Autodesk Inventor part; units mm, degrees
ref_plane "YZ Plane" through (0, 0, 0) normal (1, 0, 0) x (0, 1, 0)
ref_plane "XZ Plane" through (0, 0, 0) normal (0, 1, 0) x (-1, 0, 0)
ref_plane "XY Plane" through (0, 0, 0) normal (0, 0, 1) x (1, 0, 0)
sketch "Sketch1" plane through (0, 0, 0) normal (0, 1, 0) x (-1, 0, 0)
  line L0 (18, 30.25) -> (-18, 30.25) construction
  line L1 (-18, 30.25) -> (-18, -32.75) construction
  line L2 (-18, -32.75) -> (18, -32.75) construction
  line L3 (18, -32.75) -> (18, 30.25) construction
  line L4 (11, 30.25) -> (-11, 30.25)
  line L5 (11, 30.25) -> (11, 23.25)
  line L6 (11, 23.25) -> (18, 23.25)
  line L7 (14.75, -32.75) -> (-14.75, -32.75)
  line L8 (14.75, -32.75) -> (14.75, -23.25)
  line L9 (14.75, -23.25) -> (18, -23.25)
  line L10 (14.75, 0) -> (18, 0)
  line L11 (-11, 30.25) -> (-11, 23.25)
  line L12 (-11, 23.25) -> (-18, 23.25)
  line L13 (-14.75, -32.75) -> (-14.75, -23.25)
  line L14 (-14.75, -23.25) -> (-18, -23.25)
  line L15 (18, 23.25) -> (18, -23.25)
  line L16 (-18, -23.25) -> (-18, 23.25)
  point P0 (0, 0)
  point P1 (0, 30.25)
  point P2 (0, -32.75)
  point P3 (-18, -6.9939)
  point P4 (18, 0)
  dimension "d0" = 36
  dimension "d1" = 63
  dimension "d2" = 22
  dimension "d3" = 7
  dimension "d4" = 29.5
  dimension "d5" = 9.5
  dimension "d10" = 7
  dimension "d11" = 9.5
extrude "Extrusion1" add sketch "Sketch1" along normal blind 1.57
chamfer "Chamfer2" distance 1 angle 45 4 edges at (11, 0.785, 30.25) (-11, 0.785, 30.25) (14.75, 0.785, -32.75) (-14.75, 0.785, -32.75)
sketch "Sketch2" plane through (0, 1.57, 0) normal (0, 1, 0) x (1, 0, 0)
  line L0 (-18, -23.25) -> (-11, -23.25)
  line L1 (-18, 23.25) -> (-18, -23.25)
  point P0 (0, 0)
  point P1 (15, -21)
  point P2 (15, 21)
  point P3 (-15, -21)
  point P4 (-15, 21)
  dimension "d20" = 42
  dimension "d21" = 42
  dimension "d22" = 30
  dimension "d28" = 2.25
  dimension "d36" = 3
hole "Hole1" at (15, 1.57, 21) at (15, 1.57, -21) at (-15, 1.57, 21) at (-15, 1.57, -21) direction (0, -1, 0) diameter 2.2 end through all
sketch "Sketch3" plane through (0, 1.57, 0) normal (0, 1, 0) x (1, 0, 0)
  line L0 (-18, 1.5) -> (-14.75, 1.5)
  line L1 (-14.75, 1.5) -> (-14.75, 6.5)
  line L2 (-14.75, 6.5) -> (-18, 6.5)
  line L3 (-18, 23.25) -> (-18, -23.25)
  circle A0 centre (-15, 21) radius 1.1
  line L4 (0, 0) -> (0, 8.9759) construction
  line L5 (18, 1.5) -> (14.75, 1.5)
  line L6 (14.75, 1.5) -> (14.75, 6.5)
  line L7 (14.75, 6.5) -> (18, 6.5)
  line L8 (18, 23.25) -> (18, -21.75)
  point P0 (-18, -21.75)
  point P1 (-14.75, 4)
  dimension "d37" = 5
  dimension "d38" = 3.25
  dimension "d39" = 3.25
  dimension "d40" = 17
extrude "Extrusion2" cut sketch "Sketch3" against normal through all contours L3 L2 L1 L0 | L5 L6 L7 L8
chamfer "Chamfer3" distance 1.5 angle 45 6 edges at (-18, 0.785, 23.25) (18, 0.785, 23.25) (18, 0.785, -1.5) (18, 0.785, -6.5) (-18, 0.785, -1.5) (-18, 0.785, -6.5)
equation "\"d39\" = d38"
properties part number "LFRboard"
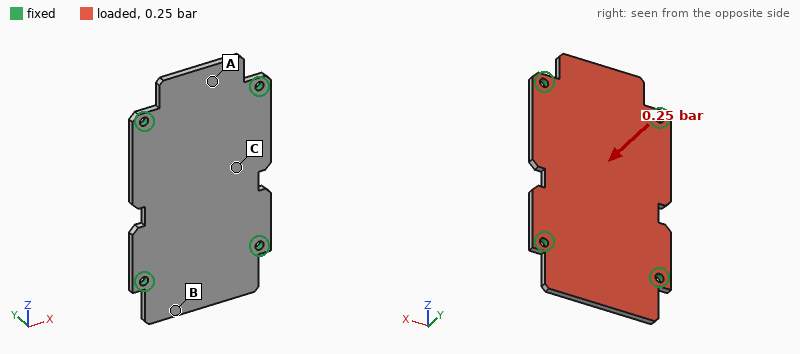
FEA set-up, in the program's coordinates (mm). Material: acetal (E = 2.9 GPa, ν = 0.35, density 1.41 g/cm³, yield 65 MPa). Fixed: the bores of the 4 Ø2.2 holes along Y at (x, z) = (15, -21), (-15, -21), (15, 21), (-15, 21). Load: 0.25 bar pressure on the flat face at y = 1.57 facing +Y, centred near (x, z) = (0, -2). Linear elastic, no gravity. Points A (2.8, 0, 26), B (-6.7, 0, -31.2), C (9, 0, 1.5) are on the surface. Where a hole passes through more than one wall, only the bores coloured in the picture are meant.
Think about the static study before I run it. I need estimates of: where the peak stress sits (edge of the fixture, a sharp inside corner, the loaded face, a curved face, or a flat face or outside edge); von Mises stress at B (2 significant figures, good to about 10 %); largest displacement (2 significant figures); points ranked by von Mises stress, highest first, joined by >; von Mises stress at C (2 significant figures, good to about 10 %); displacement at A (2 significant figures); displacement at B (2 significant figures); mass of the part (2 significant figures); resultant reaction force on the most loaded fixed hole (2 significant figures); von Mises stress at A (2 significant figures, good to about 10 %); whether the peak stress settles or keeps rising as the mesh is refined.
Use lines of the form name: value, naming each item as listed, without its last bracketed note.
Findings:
where the peak stress sits: edge of the fixture
von Mises stress at B: 1.4 MPa
largest displacement: 0.31 mm
points ranked by von Mises stress, highest first, joined by >: C > A > B
von Mises stress at C: 4.5 MPa
displacement at A: 0.061 mm
displacement at B: 0.073 mm
mass of the part: 4.5 g
resultant reaction force on the most loaded fixed hole: 14 N
von Mises stress at A: 2.8 MPa
whether the peak stress settles or keeps rising as the mesh is refined: keeps rising
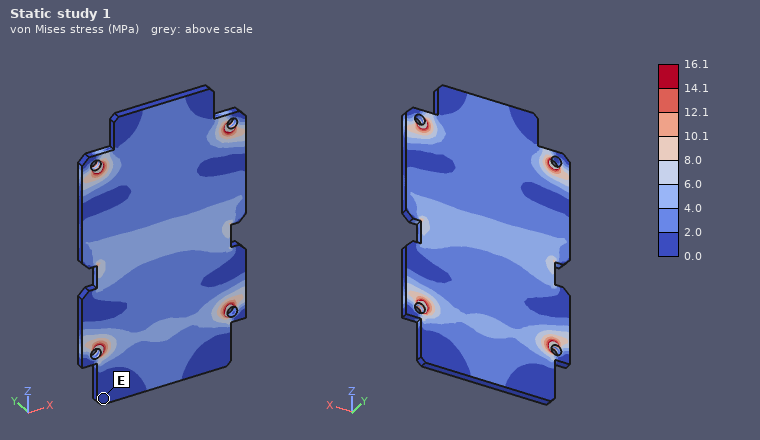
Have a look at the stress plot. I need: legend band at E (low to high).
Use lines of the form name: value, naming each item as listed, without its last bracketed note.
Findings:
legend band at E: 0.0 to 2.0 MPa
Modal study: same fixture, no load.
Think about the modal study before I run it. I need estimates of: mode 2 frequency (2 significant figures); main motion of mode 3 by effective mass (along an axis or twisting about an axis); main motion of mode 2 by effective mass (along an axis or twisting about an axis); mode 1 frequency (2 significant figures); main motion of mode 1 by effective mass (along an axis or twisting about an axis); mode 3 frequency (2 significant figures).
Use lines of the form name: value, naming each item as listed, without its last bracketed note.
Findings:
mode 2 frequency: 1600 Hz
main motion of mode 3 by effective mass: twisting about Z
main motion of mode 2 by effective mass: along Y
mode 1 frequency: 1100 Hz
main motion of mode 1 by effective mass: along Y
mode 3 frequency: 1700 Hz
